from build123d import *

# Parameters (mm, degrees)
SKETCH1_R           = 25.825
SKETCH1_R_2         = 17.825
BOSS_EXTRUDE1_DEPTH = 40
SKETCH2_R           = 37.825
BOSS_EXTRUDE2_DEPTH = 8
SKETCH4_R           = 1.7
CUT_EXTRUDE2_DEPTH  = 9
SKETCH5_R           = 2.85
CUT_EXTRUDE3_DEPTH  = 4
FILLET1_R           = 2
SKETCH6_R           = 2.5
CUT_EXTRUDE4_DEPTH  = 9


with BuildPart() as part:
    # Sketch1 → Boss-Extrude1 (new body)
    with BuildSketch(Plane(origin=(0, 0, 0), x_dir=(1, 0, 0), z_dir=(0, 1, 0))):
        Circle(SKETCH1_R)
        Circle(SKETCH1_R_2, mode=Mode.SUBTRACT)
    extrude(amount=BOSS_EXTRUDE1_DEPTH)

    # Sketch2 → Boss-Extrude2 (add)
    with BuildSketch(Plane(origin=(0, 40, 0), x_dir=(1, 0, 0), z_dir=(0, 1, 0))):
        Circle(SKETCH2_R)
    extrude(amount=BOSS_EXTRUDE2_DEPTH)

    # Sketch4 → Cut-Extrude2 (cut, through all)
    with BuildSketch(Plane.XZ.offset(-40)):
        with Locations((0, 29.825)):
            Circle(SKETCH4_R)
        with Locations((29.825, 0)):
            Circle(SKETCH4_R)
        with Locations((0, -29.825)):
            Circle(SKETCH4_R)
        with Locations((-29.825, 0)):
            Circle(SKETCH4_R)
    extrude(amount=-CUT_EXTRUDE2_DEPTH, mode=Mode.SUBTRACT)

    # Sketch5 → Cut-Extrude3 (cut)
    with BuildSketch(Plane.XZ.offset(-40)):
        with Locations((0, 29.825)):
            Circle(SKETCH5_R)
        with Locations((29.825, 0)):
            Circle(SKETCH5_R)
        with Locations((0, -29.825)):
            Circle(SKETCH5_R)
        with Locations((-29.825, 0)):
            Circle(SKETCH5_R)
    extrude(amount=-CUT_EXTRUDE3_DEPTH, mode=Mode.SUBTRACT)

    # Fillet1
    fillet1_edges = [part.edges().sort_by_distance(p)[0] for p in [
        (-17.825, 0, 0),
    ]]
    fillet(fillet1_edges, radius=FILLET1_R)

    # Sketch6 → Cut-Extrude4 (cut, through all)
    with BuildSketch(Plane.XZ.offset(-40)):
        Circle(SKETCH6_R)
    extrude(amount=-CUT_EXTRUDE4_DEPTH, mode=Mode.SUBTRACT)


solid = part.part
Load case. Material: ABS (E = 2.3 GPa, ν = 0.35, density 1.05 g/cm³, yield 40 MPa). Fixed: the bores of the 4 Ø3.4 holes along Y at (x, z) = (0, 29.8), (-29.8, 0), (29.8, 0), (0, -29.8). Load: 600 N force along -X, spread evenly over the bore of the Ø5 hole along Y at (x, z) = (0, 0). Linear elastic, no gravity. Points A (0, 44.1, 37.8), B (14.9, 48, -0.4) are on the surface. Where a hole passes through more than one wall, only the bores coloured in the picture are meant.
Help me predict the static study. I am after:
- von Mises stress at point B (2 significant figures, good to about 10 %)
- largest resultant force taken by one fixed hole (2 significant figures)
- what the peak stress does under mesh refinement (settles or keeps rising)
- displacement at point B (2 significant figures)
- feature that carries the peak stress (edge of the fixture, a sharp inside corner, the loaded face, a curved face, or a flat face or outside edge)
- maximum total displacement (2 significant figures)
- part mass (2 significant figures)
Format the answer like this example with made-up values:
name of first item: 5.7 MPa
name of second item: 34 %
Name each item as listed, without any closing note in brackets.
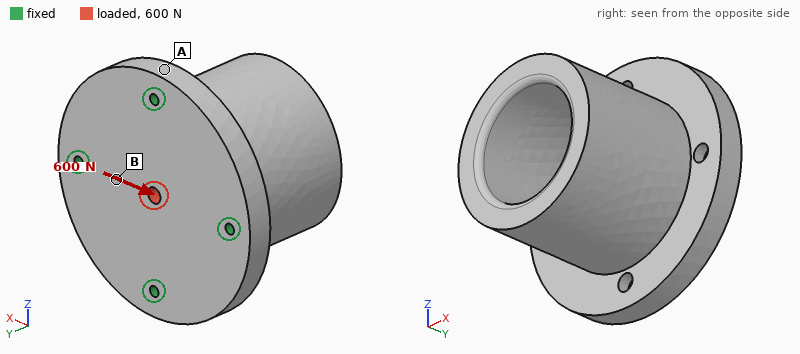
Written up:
von Mises stress at point B: 1.9 MPa
largest resultant force taken by one fixed hole: 180 N
what the peak stress does under mesh refinement: keeps rising
displacement at point B: 15 µm
feature that carries the peak stress: edge of the fixture
maximum total displacement: 31 µm
part mass: 83 g
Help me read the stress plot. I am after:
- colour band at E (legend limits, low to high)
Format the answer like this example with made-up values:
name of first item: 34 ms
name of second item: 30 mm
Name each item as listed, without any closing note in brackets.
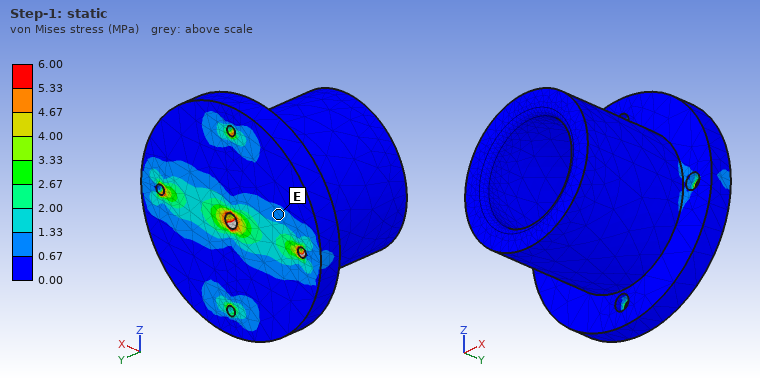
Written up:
colour band at E: 0.67 to 1.33 MPa
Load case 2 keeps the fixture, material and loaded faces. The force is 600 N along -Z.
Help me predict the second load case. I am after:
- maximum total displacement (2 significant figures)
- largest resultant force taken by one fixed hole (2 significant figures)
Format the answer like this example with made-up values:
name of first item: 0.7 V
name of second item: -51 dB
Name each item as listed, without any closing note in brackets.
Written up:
maximum total displacement: 31 µm
largest resultant force taken by one fixed hole: 180 N
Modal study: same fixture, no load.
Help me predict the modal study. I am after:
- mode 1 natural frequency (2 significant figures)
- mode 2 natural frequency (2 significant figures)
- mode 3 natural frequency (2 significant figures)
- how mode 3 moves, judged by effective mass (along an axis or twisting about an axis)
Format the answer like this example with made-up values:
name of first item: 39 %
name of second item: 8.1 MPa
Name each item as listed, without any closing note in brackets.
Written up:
mode 1 natural frequency: 2000 Hz
mode 2 natural frequency: 2000 Hz
mode 3 natural frequency: 2900 Hz
how mode 3 moves, judged by effective mass: along Y
